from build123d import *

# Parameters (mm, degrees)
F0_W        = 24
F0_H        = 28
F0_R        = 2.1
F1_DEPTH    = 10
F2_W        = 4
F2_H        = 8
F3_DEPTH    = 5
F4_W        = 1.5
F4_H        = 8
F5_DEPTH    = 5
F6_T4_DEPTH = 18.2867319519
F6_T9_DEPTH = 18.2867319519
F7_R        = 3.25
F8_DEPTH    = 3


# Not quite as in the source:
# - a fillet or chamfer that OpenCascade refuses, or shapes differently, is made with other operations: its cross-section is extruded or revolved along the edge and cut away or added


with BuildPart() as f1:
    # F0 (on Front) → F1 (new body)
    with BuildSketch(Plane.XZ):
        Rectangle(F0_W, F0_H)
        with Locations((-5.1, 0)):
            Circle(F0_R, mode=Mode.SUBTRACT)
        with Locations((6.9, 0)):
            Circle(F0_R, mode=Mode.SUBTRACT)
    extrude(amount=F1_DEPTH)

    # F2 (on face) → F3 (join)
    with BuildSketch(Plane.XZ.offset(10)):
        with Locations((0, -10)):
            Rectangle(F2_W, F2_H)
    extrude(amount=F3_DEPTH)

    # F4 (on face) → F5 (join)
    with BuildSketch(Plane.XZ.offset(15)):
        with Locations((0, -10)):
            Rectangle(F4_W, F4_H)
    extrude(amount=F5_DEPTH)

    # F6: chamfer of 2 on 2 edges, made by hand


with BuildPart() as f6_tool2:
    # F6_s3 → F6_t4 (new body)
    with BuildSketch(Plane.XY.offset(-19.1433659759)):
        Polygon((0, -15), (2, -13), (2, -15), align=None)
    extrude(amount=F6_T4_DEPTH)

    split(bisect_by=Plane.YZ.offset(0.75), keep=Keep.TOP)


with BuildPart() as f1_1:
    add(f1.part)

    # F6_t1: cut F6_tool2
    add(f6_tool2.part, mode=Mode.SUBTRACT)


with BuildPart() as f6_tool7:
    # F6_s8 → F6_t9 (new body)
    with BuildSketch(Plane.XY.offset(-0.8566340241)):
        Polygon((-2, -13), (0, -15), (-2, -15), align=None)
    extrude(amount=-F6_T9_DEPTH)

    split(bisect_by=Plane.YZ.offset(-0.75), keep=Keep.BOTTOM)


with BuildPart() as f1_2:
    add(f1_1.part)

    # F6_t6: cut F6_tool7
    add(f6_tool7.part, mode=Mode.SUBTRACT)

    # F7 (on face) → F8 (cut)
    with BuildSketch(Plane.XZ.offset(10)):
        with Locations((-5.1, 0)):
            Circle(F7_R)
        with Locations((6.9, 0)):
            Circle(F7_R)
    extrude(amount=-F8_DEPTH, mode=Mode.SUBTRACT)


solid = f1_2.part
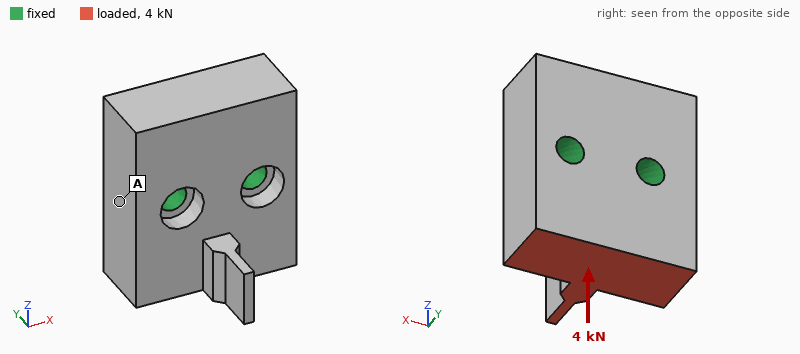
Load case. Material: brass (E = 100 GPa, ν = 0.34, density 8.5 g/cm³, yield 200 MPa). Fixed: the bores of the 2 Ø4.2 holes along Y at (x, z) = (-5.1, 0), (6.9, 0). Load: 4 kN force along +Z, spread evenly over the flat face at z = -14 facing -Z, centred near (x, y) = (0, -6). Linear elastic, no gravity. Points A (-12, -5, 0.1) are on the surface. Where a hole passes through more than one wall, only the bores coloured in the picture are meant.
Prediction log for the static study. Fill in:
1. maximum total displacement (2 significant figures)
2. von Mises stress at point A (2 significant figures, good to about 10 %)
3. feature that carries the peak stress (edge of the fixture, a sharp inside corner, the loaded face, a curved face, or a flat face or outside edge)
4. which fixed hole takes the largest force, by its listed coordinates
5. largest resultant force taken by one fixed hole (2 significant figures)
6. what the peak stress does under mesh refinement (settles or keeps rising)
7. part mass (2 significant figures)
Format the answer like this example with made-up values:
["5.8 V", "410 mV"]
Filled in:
["18 µm", "10.0 MPa", "edge of the fixture", "(-5.1, 0)", "2.3 kN", "keeps rising", "55 g"]
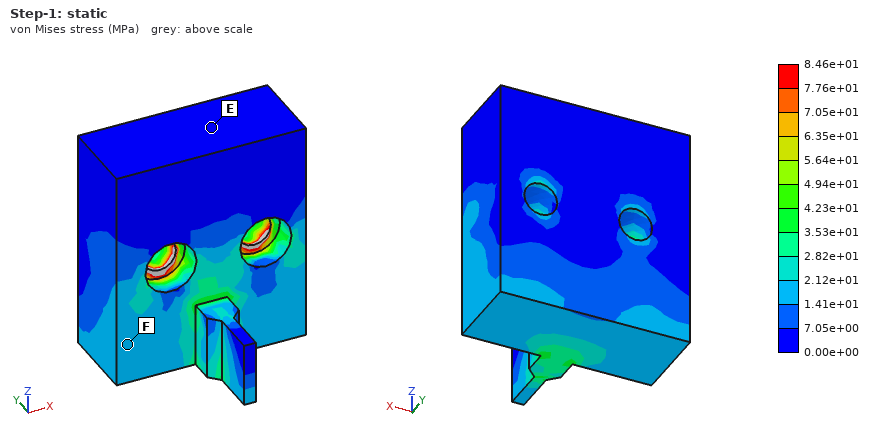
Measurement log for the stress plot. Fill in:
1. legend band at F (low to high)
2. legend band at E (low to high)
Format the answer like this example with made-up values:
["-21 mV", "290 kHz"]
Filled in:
["1.41e+01 to 2.12e+01 MPa", "0.00e+00 to 7.05e+00 MPa"]
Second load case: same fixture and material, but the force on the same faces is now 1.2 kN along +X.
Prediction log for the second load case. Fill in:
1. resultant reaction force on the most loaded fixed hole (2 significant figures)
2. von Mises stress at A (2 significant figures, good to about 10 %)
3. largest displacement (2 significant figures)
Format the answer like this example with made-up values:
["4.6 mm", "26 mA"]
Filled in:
["1.3 kN", "11 MPa", "18 µm"]
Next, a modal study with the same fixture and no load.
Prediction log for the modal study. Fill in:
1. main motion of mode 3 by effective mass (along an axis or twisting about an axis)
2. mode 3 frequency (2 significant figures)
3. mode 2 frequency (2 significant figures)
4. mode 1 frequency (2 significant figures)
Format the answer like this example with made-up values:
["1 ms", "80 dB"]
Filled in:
["along Y", "20 kHz", "17 kHz", "14 kHz"]
